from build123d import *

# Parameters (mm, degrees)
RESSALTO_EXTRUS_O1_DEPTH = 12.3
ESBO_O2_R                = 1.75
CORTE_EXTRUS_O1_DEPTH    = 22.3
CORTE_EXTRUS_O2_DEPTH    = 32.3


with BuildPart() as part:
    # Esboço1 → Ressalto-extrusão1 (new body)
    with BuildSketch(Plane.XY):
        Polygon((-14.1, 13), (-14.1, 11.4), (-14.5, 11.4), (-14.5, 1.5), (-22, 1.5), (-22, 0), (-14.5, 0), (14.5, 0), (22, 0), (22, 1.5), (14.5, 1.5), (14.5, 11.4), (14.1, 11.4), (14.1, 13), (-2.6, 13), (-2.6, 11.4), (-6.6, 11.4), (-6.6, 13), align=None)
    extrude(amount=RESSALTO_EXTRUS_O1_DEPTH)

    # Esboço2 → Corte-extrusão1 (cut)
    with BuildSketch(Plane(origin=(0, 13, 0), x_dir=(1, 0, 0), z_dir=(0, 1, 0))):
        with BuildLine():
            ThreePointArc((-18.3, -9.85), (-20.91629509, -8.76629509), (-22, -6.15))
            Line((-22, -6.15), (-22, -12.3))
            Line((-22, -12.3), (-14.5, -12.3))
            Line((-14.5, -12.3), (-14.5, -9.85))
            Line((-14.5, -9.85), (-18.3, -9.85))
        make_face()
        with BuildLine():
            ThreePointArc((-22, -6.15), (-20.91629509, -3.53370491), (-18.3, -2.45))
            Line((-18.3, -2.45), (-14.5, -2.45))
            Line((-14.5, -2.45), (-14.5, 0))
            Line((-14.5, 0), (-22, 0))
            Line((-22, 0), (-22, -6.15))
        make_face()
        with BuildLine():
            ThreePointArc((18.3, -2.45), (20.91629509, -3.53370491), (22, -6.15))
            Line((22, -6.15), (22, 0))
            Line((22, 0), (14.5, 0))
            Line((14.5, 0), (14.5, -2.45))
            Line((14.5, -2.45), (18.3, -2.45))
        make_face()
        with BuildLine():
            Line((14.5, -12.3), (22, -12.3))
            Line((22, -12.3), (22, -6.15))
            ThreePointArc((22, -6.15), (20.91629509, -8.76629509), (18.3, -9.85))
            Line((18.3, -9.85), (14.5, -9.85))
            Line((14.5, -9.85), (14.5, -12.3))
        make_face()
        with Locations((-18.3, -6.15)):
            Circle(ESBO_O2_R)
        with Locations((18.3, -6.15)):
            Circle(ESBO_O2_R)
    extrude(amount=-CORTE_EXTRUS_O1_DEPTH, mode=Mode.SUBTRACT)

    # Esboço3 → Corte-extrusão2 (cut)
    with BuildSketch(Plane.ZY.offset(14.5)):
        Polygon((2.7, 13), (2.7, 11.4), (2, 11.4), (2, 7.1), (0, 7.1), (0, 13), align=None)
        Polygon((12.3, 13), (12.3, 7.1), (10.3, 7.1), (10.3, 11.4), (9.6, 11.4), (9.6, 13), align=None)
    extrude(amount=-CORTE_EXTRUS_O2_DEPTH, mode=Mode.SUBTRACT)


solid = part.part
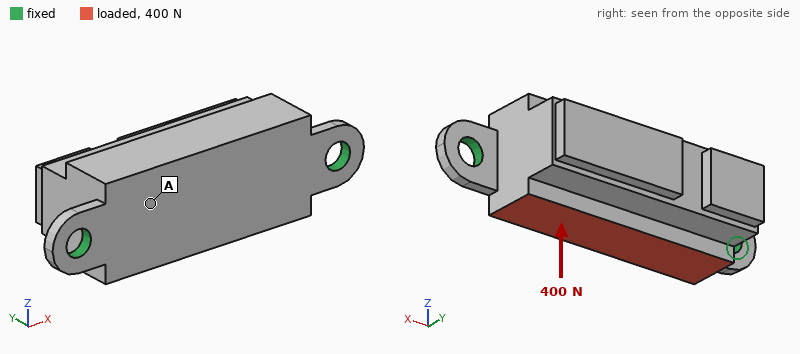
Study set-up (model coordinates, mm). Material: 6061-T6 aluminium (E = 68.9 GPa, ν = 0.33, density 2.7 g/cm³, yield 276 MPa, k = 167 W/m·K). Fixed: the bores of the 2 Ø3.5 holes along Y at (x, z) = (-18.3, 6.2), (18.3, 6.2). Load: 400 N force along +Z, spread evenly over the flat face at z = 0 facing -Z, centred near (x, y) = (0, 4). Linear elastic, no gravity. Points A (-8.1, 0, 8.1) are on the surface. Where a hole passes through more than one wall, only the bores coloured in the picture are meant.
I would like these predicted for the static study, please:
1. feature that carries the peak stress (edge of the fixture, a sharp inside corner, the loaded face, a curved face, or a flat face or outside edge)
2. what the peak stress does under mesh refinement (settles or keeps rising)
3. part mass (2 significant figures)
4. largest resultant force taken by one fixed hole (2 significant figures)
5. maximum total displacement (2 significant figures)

edge of the fixture
keeps rising
11 g
200 N
63 µm
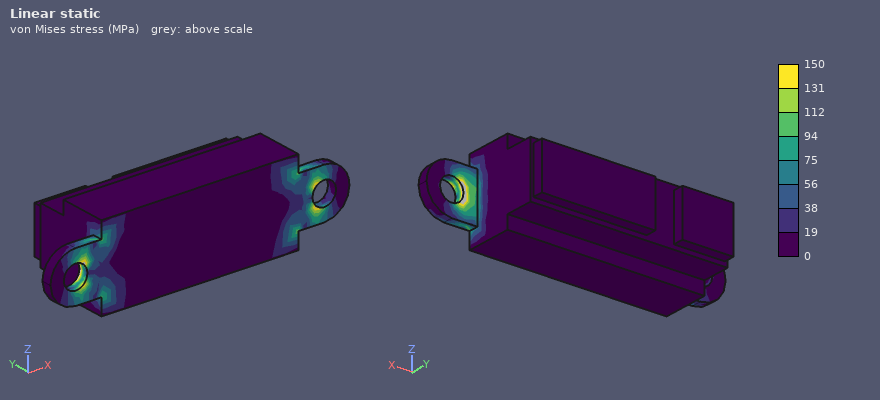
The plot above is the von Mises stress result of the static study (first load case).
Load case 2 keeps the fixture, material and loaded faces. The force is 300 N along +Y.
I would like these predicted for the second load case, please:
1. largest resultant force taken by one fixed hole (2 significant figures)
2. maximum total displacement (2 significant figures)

180 N
97 µm
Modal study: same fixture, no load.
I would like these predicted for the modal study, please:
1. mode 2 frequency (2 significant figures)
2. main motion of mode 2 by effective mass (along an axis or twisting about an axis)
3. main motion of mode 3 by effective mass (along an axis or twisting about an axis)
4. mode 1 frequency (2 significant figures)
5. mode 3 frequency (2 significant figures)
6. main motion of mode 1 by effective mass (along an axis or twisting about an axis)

11 kHz
along Y
along X
3500 Hz
17 kHz
along Z
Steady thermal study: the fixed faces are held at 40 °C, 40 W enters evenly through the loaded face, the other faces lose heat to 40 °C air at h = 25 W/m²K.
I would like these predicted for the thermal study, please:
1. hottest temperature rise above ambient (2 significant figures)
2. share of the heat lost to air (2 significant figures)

53 K
4.4 %
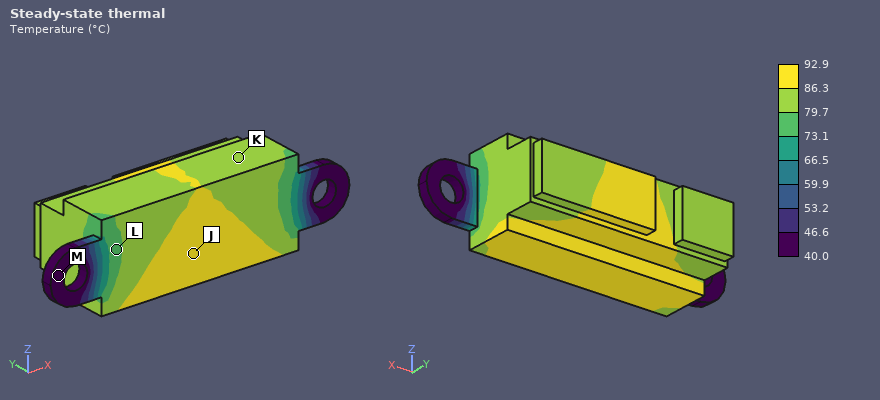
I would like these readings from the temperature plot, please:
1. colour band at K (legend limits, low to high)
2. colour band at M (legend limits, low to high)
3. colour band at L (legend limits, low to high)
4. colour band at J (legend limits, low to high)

79.7 to 86.3 °C
40.0 to 46.6 °C
73.1 to 79.7 °C
86.3 to 92.9 °C
